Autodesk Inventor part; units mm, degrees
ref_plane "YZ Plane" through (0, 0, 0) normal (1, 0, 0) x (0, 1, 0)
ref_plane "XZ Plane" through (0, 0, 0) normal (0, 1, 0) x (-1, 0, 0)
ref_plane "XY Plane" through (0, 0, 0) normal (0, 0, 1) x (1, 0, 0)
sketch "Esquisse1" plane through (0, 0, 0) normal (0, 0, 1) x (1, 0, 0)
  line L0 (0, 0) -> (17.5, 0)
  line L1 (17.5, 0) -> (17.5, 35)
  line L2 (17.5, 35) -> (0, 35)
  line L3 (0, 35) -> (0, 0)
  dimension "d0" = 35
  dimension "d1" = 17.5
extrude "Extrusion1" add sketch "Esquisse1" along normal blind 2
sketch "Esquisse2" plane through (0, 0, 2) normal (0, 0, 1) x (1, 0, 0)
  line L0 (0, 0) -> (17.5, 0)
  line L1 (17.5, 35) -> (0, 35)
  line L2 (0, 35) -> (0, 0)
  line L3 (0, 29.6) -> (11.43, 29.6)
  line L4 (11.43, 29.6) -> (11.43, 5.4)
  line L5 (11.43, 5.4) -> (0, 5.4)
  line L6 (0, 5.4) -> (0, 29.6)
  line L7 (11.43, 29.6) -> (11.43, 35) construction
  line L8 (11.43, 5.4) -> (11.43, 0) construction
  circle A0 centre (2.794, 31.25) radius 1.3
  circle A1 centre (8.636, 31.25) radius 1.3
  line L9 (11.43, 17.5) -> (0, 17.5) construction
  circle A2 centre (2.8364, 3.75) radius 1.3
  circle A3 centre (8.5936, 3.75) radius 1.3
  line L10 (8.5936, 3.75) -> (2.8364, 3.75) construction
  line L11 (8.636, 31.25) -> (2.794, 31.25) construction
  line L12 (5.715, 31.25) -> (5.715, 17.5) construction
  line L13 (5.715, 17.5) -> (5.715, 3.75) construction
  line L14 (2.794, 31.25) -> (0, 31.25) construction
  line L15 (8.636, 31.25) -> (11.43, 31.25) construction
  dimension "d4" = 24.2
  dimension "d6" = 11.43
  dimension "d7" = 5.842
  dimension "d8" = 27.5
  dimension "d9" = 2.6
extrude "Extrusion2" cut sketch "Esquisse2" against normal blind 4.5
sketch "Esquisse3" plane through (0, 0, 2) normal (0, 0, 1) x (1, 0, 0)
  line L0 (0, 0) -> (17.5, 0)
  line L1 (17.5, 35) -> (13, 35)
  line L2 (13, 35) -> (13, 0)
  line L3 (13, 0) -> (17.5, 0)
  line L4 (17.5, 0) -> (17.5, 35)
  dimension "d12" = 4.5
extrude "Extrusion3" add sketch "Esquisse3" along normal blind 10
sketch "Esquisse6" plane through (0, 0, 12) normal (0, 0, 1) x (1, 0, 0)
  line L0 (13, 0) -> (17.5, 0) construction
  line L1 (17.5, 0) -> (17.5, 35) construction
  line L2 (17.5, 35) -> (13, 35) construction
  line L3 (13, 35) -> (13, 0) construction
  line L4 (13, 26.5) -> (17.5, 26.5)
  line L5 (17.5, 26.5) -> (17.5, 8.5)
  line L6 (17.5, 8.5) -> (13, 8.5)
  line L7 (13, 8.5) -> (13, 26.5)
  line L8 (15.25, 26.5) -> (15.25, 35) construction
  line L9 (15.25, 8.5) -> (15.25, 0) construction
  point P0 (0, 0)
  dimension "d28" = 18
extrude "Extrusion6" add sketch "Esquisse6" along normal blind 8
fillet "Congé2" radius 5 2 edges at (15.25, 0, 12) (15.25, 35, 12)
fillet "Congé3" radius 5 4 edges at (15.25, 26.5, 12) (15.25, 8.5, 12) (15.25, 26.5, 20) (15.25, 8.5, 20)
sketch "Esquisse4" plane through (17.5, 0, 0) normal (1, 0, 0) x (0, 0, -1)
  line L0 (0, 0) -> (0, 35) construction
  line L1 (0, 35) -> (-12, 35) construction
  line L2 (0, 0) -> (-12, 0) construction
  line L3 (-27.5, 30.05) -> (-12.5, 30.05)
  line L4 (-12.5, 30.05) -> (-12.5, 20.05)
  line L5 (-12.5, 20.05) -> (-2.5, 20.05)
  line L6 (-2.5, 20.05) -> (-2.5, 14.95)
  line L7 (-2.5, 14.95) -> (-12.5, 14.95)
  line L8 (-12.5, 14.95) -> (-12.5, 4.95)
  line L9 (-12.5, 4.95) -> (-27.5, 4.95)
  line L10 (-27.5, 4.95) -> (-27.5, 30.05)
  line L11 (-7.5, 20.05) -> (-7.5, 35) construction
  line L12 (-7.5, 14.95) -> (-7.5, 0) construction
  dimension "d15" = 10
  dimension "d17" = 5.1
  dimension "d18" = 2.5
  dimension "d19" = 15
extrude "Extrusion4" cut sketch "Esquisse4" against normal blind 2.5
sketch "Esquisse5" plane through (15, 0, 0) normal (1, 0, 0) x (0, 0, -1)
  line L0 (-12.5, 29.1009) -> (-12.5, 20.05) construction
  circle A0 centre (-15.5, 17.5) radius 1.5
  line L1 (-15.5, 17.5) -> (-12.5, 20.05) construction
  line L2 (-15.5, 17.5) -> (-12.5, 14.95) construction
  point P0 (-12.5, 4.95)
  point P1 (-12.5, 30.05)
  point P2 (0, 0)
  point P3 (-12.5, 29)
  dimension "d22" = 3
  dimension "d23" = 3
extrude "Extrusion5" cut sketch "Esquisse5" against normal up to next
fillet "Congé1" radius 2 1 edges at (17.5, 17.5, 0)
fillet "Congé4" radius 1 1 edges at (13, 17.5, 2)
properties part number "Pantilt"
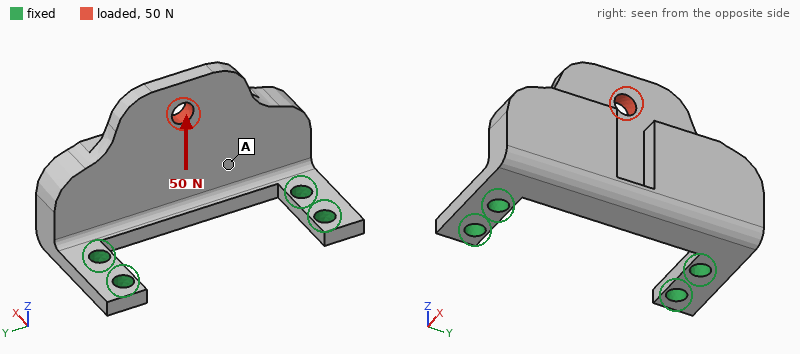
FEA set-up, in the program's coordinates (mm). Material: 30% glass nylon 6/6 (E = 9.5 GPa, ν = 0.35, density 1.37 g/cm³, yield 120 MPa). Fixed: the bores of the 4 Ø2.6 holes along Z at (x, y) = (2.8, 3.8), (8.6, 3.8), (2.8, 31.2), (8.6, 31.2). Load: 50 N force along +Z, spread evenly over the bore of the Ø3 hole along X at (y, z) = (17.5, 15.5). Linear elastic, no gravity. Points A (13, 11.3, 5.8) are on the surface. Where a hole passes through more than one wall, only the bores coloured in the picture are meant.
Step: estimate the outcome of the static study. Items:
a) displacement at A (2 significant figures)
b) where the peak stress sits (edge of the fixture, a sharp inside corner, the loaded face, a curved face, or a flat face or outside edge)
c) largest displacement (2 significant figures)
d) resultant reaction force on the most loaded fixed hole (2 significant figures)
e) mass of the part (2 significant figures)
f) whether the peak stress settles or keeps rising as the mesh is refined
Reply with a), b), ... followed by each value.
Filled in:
a) 0.040 mm
b) edge of the fixture
c) 0.13 mm
d) 27 N
e) 3.2 g
f) keeps rising
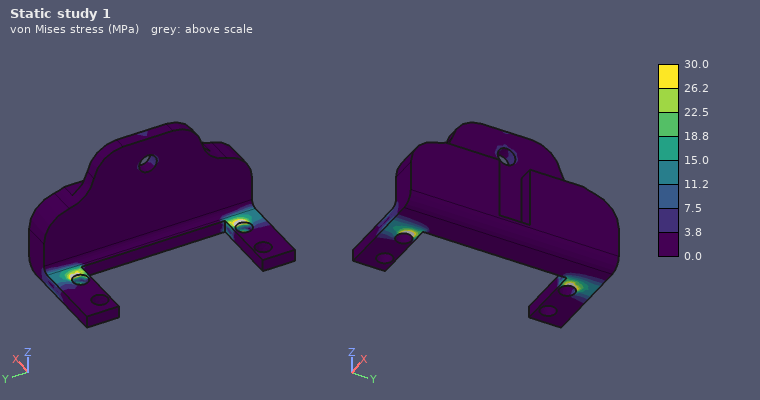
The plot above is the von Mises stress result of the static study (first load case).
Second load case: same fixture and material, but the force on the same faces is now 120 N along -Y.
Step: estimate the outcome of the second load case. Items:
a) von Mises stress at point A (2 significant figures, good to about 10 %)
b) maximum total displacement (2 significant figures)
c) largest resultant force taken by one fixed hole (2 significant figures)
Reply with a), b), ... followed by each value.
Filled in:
a) 6.3 MPa
b) 64 µm
c) 91 N
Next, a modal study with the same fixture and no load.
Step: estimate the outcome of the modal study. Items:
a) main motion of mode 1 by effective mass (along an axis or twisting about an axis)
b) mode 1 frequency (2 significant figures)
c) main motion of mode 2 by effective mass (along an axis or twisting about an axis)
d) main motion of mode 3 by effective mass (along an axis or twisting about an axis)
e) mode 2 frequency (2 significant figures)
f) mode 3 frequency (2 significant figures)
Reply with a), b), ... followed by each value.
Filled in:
a) along X
b) 1400 Hz
c) along Y
d) along Z
e) 5600 Hz
f) 6800 Hz
